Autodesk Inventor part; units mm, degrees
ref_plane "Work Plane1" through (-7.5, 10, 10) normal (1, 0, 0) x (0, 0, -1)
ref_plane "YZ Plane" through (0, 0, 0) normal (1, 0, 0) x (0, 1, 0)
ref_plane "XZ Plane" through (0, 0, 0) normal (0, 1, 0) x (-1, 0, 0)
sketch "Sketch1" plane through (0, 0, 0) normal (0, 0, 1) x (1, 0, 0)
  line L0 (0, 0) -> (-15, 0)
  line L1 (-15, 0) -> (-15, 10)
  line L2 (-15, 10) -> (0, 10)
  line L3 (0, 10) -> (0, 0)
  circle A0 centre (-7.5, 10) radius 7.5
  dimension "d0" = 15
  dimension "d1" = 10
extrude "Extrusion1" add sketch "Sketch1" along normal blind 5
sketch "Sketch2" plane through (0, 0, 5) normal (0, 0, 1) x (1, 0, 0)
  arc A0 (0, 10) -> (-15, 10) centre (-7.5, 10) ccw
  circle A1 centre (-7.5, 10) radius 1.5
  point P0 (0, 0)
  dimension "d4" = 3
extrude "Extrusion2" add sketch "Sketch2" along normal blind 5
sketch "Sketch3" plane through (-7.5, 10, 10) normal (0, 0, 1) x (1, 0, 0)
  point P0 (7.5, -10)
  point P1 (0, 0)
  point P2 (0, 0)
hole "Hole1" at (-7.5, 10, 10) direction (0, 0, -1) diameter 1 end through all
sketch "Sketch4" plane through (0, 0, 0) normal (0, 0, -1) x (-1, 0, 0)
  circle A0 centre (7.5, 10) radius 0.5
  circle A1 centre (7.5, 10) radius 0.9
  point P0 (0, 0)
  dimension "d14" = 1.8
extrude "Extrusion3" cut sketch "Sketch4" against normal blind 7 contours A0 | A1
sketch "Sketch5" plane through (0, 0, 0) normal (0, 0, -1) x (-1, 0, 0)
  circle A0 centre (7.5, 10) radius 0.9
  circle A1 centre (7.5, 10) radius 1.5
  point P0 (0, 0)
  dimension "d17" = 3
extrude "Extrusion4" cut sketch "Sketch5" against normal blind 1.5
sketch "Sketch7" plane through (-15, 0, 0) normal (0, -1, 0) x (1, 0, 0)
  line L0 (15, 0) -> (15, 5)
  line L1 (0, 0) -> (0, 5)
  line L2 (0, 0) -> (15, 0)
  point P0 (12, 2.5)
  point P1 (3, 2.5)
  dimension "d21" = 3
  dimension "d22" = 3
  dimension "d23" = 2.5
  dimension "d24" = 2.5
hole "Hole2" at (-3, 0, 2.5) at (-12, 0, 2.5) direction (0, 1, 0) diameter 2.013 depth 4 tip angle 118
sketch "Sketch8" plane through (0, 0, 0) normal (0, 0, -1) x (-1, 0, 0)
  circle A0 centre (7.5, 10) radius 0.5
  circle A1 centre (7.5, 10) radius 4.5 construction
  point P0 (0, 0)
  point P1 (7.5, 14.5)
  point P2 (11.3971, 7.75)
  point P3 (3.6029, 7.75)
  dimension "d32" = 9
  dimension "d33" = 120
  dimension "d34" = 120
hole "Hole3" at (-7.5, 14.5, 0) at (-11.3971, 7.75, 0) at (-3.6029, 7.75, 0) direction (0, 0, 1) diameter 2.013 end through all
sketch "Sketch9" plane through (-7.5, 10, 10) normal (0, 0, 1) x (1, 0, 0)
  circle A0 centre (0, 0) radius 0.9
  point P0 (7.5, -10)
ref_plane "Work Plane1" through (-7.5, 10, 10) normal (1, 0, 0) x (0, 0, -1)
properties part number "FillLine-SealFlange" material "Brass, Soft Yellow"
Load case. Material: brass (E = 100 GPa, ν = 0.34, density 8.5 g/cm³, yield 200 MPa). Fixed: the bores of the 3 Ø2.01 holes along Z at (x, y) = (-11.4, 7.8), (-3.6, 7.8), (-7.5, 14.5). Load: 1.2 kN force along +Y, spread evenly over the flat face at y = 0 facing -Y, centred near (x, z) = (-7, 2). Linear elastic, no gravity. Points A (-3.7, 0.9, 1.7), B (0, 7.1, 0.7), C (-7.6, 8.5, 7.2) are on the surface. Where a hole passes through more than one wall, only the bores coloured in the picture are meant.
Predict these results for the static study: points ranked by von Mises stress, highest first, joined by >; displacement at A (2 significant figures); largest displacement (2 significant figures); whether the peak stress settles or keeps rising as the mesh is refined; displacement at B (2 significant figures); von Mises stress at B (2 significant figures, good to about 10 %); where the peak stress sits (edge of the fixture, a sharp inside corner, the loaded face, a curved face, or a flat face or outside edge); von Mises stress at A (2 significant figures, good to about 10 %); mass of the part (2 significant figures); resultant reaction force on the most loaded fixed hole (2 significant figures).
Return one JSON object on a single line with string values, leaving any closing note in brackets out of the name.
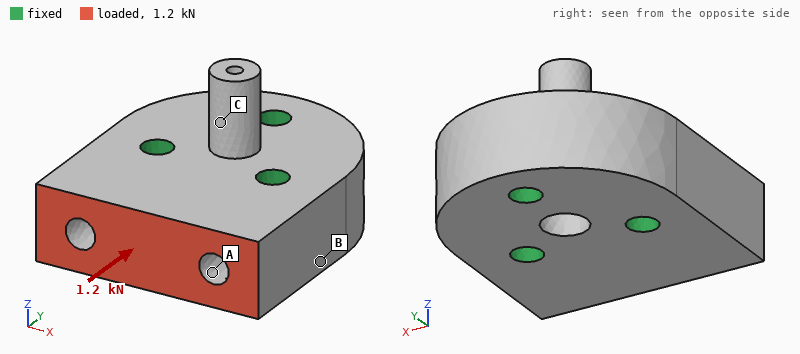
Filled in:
{"points ranked by von Mises stress, highest first, joined by >": "A > B > C", "displacement at A": "1.3 µm", "largest displacement": "1.6 µm", "whether the peak stress settles or keeps rising as the mesh is refined": "keeps rising", "displacement at B": "0.57 µm", "von Mises stress at B": "11 MPa", "where the peak stress sits": "edge of the fixture", "von Mises stress at A": "18 MPa", "mass of the part": "9.6 g", "resultant reaction force on the most loaded fixed hole": "570 N"}
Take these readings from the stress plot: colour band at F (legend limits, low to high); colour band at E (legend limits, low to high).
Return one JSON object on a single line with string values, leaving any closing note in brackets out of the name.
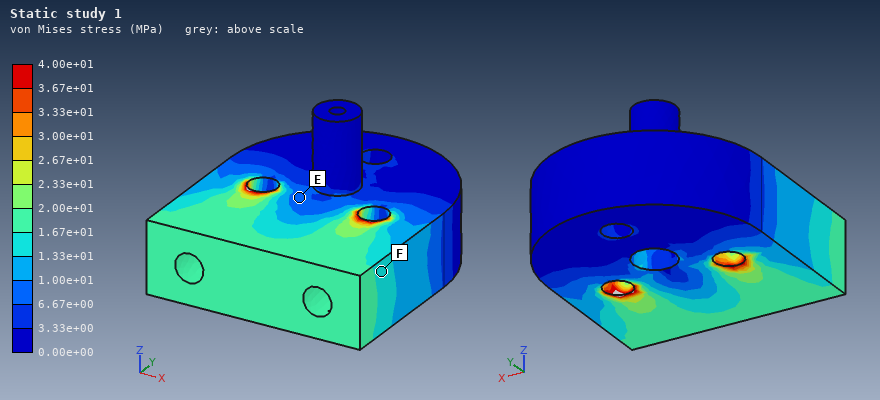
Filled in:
{"colour band at F": "1.33e+01 to 1.67e+01 MPa", "colour band at E": "6.67e+00 to 1.00e+01 MPa"}
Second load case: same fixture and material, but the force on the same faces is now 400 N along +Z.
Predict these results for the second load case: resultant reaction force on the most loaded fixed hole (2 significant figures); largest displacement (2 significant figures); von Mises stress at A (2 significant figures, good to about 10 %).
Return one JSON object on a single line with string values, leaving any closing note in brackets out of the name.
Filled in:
{"resultant reaction force on the most loaded fixed hole": "230 N", "largest displacement": "6.2 µm", "von Mises stress at A": "22 MPa"}
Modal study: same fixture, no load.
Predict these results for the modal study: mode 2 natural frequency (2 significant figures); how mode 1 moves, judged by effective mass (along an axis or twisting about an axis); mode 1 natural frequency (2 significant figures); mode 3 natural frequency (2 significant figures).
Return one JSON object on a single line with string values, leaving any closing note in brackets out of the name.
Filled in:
{"mode 2 natural frequency": "38 kHz", "how mode 1 moves, judged by effective mass": "along Z", "mode 1 natural frequency": "36 kHz", "mode 3 natural frequency": "38 kHz"}
